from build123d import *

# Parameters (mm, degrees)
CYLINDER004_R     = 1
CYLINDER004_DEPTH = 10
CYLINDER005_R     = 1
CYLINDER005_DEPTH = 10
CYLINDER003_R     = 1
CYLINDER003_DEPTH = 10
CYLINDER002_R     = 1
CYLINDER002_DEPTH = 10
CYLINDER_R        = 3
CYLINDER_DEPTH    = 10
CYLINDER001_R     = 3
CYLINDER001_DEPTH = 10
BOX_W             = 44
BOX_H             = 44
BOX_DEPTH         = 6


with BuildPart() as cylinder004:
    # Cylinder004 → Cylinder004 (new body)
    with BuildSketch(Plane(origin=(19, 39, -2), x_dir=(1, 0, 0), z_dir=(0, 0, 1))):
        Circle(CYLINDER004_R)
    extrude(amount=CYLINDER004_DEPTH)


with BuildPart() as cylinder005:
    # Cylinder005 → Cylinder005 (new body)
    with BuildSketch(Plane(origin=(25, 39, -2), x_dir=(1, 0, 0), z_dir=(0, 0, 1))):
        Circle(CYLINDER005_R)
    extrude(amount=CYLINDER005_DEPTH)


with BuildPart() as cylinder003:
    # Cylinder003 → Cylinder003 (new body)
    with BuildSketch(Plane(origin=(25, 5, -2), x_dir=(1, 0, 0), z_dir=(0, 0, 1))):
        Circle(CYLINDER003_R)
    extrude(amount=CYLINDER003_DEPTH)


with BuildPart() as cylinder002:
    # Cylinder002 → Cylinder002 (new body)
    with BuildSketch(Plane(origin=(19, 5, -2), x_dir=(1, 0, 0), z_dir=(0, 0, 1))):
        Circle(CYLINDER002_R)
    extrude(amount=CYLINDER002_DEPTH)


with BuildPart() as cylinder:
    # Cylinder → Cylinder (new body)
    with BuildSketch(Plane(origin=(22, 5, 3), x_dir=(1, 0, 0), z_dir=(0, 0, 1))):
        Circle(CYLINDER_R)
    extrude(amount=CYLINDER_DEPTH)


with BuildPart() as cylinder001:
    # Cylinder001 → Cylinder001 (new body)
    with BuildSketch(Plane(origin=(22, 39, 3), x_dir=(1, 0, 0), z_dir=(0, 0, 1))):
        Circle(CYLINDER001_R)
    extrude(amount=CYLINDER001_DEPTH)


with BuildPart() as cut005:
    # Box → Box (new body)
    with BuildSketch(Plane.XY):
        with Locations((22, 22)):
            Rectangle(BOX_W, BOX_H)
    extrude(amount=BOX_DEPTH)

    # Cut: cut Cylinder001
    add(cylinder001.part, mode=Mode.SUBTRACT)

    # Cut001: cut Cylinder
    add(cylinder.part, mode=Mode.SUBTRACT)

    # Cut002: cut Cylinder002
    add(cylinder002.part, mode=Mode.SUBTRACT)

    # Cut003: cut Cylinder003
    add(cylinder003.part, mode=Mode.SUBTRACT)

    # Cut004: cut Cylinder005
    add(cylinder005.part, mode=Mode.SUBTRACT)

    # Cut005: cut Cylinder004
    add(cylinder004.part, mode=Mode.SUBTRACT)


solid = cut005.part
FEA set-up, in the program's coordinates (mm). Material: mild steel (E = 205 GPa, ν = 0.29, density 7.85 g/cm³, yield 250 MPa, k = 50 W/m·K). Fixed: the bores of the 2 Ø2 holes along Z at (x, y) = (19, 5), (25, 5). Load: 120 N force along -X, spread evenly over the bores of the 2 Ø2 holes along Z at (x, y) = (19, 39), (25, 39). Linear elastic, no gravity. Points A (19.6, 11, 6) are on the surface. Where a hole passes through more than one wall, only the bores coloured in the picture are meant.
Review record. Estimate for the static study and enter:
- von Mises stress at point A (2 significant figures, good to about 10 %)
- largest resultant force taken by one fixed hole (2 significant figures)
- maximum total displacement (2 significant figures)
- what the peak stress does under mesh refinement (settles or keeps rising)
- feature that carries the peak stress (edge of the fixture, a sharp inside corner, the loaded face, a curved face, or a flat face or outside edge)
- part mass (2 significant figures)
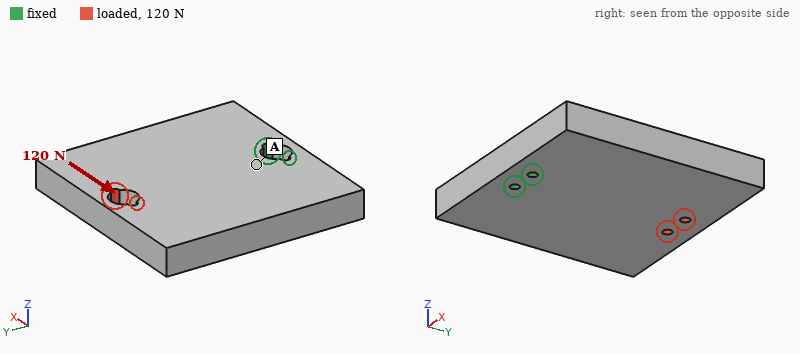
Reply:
8.0 MPa
500 N
5.6 µm
keeps rising
edge of the fixture
89 g
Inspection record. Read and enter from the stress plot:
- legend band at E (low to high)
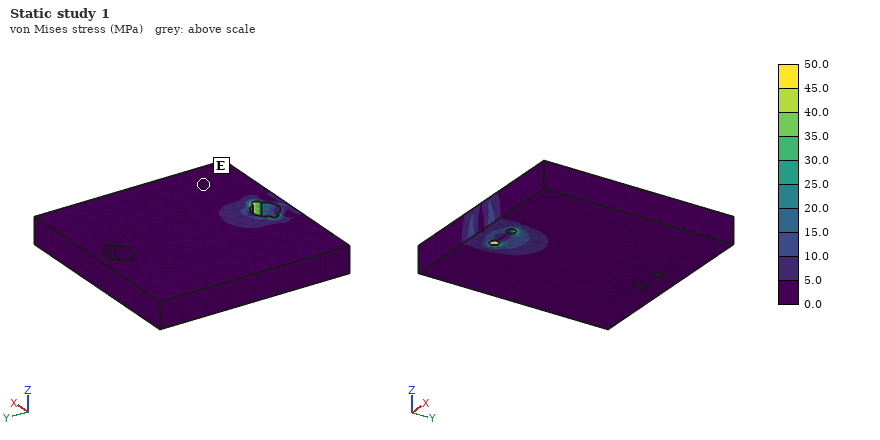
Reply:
0.0 to 5.0 MPa
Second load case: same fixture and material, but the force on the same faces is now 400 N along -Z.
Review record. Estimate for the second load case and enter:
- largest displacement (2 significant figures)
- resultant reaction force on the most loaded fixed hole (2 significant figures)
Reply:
70 µm
200 N
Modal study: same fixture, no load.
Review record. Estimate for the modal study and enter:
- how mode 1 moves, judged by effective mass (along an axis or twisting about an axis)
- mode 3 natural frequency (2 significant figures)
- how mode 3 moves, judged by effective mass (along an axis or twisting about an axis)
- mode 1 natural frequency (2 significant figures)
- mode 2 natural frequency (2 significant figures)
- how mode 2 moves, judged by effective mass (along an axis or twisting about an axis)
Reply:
along Z
4400 Hz
twisting about Y
2400 Hz
3900 Hz
along X
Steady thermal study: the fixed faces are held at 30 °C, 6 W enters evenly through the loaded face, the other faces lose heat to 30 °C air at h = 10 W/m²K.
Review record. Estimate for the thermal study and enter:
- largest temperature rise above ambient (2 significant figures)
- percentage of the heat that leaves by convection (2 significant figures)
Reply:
24 K
9.3 %
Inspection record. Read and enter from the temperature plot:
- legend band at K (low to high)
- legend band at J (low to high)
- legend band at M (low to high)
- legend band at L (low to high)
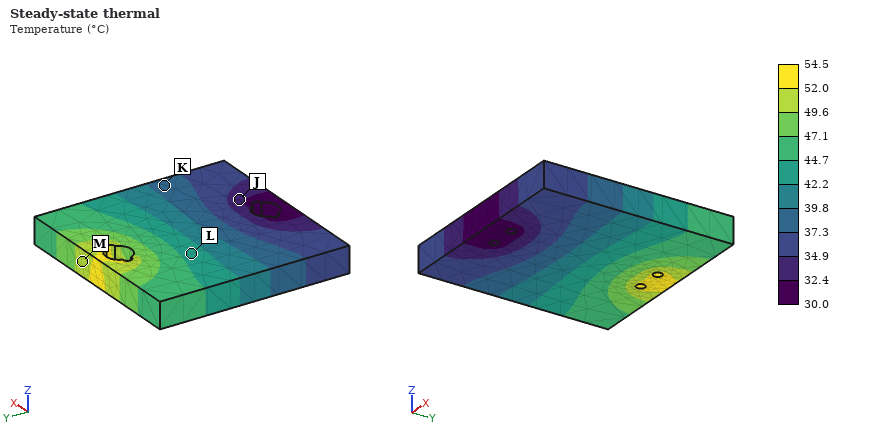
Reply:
37.3 to 39.8 °C
32.4 to 34.9 °C
49.6 to 52.0 °C
42.2 to 44.7 °C
